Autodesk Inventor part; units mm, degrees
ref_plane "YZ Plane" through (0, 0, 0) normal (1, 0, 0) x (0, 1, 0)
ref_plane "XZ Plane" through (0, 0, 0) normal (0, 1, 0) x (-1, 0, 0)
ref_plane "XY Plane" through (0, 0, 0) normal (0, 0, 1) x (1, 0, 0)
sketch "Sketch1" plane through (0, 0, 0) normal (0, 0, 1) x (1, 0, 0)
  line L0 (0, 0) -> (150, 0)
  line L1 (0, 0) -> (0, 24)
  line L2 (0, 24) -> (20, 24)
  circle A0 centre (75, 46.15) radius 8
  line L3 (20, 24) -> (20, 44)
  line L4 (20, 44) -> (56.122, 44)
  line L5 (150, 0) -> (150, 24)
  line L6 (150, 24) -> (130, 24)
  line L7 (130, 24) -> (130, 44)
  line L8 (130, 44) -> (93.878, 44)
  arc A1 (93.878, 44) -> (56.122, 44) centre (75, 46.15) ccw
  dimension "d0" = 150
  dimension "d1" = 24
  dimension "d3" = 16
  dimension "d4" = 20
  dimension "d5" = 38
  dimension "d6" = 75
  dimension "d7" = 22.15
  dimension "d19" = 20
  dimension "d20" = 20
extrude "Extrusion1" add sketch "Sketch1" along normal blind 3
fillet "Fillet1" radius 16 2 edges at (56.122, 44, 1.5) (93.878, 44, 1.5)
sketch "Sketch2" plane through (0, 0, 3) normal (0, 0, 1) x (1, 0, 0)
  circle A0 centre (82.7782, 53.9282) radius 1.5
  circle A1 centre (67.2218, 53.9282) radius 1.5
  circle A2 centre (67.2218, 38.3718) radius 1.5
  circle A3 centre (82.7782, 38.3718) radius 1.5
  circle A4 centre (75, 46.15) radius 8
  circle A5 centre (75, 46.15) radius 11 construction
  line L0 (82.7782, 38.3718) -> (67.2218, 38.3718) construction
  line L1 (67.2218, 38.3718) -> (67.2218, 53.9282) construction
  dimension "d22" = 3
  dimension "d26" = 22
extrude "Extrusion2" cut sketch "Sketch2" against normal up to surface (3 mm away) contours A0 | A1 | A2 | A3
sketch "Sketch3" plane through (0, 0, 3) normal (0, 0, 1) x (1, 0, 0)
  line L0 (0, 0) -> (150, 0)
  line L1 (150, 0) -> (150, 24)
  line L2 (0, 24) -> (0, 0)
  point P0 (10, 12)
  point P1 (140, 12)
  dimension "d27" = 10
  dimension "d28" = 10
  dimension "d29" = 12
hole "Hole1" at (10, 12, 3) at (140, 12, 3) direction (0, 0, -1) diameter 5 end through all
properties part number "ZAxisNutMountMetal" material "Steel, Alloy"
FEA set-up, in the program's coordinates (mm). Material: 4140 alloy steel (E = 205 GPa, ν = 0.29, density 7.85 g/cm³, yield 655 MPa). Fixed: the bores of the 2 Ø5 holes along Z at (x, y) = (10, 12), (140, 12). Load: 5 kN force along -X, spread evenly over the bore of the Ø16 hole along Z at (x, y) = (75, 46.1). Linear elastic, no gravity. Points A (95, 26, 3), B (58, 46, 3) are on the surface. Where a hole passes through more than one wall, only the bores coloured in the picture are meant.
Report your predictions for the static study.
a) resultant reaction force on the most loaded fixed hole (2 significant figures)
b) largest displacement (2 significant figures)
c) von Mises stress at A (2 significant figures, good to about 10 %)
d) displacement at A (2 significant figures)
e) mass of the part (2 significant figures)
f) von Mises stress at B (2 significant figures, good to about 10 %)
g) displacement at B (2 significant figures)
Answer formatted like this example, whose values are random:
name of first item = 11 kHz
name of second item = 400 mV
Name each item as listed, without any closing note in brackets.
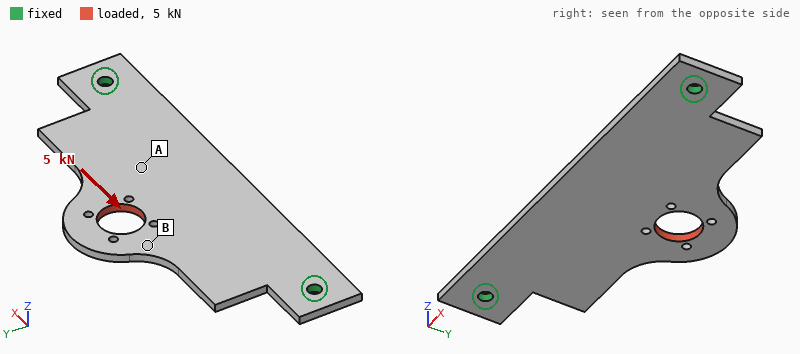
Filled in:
resultant reaction force on the most loaded fixed hole = 2.8 kN
largest displacement = 25 µm
von Mises stress at A = 18 MPa
displacement at A = 8.3 µm
mass of the part = 150 g
von Mises stress at B = 58 MPa
displacement at B = 16 µm
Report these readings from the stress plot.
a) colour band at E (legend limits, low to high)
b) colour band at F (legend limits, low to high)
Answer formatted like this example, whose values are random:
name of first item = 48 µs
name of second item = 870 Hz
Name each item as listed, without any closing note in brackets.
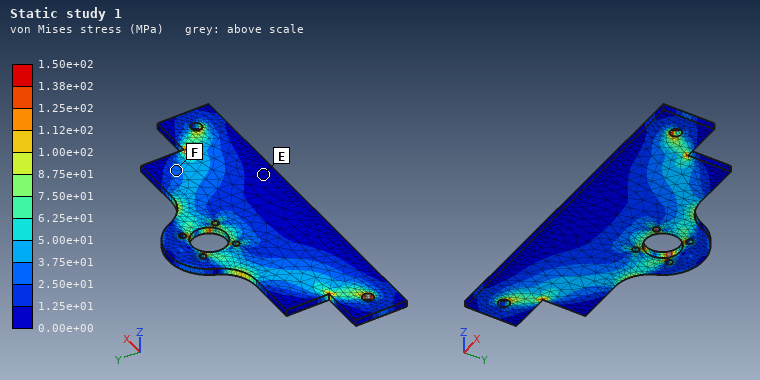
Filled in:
colour band at E = 0.00e+00 to 1.25e+01 MPa
colour band at F = 2.50e+01 to 3.75e+01 MPa
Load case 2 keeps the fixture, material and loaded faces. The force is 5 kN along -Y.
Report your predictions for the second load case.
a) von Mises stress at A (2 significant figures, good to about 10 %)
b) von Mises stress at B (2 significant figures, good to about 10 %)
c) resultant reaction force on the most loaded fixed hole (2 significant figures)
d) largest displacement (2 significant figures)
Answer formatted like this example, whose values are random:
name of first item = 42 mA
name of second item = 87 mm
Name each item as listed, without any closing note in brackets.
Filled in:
von Mises stress at A = 39 MPa
von Mises stress at B = 56 MPa
resultant reaction force on the most loaded fixed hole = 3.3 kN
largest displacement = 48 µm
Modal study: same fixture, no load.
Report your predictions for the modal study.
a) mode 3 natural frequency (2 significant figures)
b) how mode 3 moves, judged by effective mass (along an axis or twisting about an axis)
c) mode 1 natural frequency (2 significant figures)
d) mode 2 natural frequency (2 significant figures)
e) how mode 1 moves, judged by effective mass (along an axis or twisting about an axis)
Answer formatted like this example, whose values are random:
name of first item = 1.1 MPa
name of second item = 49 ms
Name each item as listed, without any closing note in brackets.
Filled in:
mode 3 natural frequency = 1900 Hz
how mode 3 moves, judged by effective mass = twisting about Y
mode 1 natural frequency = 610 Hz
mode 2 natural frequency = 1200 Hz
how mode 1 moves, judged by effective mass = along Z
